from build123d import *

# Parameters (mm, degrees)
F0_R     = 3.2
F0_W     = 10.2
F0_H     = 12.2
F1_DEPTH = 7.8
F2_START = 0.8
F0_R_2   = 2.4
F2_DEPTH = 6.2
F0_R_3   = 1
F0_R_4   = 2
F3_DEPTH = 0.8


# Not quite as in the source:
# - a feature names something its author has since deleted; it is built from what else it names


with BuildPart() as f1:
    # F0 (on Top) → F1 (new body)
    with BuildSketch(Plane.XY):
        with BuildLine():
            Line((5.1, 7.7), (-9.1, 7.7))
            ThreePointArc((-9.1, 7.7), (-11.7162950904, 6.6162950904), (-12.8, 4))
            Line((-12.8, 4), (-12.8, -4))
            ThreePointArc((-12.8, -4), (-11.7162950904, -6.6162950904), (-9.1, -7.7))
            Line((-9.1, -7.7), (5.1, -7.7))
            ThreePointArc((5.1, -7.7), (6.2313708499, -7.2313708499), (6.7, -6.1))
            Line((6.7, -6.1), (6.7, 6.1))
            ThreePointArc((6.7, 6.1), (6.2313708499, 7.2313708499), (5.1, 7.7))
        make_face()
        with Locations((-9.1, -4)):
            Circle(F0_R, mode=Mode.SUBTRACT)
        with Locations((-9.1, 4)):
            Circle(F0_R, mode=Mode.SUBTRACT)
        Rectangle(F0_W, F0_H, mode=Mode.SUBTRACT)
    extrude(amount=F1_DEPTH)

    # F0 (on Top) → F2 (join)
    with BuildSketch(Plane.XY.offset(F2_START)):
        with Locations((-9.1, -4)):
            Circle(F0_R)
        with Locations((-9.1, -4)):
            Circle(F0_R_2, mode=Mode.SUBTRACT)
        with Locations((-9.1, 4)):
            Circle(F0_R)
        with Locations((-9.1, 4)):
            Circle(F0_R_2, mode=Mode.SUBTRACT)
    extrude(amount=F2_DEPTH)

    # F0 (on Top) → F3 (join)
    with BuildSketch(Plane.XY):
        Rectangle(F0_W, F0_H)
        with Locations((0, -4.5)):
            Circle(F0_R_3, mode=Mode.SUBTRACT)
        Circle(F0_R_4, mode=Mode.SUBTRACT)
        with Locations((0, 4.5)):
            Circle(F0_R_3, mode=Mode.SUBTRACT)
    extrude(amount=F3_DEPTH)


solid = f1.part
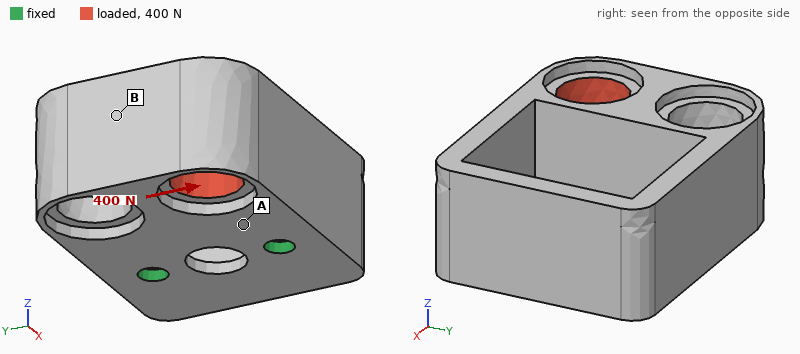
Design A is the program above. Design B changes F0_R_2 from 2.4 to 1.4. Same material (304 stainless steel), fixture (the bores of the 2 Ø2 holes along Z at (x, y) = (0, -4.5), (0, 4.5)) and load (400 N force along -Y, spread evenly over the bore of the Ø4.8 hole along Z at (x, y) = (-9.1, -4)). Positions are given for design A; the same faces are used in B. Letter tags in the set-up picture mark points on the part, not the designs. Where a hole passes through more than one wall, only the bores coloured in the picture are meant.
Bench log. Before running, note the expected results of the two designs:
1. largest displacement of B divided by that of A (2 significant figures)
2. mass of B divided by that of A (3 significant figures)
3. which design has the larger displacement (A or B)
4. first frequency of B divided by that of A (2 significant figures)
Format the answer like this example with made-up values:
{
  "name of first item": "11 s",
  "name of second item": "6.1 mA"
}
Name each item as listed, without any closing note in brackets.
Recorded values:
{
  "largest displacement of B divided by that of A": "0.88",
  "mass of B divided by that of A": "1.14",
  "which design has the larger displacement": "A",
  "first frequency of B divided by that of A": "0.91"
}
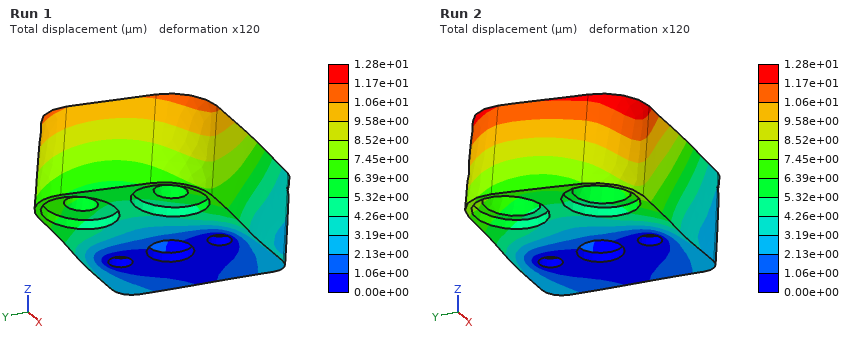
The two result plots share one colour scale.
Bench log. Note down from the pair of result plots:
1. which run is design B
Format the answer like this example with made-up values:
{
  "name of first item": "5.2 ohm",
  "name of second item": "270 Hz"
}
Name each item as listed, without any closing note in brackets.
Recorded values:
{
  "which run is design B": "Run 1"
}
